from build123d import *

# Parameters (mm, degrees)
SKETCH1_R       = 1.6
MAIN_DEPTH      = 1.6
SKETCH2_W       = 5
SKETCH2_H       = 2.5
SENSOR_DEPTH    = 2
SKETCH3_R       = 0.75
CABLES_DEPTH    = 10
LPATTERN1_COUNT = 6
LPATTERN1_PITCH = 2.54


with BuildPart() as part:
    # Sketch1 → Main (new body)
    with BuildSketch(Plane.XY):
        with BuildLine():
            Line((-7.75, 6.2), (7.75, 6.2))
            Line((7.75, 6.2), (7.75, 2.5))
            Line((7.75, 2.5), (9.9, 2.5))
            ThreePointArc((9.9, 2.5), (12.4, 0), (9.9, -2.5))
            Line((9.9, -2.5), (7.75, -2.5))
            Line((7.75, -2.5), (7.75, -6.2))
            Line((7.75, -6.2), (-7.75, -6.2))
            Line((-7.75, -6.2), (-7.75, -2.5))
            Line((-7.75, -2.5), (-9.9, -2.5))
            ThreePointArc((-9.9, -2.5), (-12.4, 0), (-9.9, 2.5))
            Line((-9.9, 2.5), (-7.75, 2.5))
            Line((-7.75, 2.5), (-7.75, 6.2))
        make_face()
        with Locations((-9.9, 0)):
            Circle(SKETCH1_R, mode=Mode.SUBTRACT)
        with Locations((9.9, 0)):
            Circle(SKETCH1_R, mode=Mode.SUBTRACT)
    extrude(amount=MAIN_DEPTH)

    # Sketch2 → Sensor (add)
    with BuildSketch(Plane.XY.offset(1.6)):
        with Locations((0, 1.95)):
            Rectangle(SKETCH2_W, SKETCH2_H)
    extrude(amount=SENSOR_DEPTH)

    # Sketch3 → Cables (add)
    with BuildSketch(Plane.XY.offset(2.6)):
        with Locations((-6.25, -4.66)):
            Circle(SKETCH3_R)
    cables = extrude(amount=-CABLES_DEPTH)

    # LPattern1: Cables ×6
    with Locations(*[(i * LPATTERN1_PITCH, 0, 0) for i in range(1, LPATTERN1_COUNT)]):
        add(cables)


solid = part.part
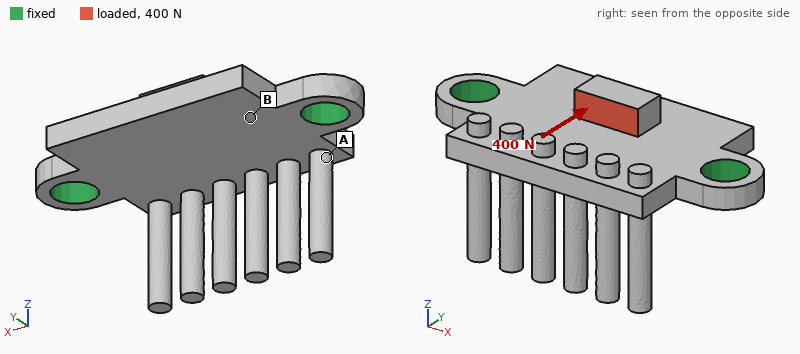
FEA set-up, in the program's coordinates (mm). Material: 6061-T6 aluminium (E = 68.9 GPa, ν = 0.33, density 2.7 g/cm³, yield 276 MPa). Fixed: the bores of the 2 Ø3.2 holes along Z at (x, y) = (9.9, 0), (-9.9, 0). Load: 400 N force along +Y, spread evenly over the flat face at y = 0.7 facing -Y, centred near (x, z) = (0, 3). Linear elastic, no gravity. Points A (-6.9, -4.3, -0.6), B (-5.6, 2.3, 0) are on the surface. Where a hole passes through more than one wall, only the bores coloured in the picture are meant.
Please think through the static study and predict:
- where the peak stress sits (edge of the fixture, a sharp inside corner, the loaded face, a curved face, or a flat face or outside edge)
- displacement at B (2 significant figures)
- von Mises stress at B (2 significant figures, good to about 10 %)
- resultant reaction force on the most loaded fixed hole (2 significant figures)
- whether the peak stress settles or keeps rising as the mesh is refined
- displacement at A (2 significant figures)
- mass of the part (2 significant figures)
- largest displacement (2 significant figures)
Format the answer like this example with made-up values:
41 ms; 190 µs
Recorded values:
edge of the fixture; 11 µm; 58 MPa; 200 N; keeps rising; 16 µm; 1.2 g; 54 µm
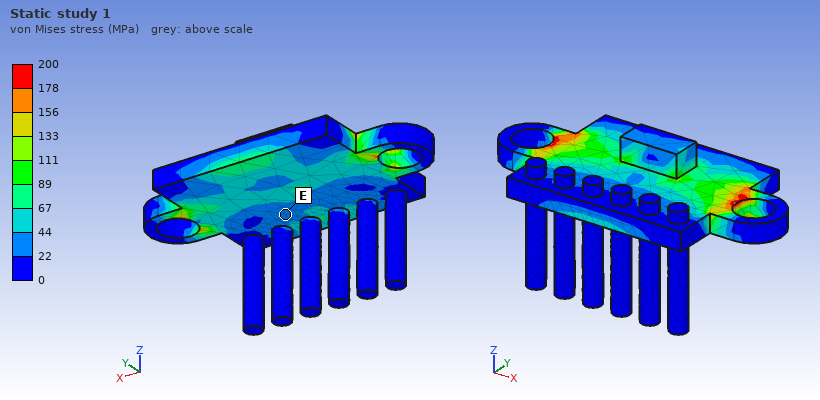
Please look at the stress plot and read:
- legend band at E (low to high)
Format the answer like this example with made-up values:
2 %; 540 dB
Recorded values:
22 to 44 MPa
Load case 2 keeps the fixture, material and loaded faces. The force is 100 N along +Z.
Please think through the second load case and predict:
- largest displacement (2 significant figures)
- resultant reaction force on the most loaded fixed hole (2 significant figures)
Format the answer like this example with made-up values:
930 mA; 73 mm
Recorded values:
14 µm; 51 N
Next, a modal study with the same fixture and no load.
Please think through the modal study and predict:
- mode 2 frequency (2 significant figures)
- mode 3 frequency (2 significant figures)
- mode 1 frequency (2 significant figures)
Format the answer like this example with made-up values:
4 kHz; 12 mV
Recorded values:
14 kHz; 15 kHz; 10 kHz
